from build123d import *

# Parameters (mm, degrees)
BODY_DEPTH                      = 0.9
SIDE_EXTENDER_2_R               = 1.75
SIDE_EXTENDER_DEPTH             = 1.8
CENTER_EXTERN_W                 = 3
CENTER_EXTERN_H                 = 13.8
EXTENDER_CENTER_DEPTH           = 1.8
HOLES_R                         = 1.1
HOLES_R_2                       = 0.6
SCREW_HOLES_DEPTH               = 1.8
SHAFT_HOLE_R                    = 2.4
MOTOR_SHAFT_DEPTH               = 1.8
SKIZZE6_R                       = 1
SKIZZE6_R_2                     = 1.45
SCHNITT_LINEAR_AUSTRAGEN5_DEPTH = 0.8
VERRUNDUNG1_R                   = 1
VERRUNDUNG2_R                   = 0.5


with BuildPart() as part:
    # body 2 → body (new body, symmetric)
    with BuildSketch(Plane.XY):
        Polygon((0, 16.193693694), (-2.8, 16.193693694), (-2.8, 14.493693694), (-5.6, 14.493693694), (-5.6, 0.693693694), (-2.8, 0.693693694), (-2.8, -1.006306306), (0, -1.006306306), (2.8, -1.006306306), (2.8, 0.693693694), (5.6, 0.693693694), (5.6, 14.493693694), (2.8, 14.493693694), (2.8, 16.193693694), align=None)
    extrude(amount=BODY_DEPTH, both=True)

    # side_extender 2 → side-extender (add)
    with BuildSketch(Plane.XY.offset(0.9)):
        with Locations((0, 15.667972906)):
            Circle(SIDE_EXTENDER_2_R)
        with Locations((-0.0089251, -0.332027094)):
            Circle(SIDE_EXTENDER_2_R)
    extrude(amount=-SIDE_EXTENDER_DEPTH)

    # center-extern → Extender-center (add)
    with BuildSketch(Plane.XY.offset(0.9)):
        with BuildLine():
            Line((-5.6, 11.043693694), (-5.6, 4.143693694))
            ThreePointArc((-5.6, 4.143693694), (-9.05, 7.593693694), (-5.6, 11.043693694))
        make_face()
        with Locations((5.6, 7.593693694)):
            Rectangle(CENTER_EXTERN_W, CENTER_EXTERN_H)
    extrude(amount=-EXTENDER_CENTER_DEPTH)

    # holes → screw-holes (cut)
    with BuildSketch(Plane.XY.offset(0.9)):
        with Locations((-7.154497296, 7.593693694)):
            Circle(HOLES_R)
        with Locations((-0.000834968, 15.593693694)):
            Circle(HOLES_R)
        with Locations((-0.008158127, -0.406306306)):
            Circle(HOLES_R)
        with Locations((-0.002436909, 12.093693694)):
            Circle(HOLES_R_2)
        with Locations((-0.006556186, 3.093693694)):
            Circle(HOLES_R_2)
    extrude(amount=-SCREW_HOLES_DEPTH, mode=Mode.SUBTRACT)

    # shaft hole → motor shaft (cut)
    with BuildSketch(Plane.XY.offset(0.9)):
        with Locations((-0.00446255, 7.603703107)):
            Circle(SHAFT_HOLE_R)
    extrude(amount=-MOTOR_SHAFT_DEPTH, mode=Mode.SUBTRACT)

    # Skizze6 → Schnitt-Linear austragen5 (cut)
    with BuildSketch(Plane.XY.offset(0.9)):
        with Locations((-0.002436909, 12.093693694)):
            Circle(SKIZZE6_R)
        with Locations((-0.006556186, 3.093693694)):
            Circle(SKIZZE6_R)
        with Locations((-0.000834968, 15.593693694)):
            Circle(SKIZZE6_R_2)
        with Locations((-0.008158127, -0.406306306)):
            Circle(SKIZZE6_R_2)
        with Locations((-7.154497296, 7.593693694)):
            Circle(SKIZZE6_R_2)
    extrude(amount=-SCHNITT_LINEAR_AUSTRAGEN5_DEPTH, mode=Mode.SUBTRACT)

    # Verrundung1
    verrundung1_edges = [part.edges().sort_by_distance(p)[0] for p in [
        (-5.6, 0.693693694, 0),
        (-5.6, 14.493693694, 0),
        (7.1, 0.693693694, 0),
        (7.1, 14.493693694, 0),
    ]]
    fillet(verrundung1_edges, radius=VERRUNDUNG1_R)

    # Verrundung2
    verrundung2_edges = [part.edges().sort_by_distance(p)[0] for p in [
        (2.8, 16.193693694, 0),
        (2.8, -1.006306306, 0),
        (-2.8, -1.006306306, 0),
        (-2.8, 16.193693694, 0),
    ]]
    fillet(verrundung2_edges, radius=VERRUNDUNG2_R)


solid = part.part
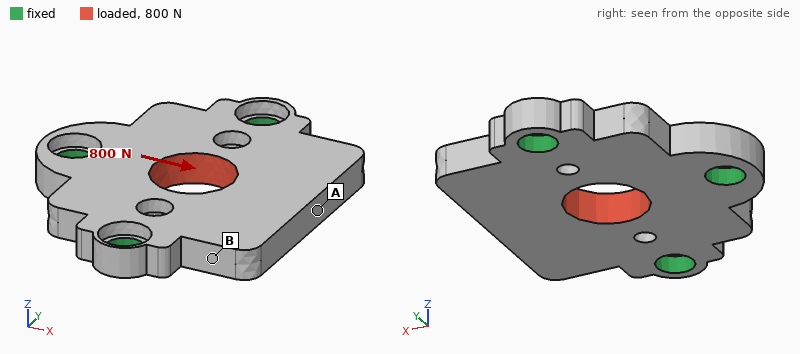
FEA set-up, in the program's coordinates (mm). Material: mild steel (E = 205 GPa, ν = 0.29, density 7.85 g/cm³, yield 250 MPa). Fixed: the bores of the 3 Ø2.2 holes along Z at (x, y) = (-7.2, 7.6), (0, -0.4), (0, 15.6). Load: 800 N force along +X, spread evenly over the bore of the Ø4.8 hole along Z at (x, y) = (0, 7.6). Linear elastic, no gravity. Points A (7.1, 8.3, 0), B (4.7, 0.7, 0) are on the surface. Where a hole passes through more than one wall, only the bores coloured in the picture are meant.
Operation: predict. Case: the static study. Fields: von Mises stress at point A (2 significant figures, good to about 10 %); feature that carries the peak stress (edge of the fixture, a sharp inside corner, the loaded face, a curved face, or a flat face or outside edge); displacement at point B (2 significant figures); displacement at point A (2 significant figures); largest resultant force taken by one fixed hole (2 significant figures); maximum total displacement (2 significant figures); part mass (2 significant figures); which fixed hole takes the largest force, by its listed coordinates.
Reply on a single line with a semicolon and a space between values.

42 MPa; edge of the fixture; 1.6 µm; 3.3 µm; 400 N; 3.5 µm; 2.5 g; (-7.2, 7.6)
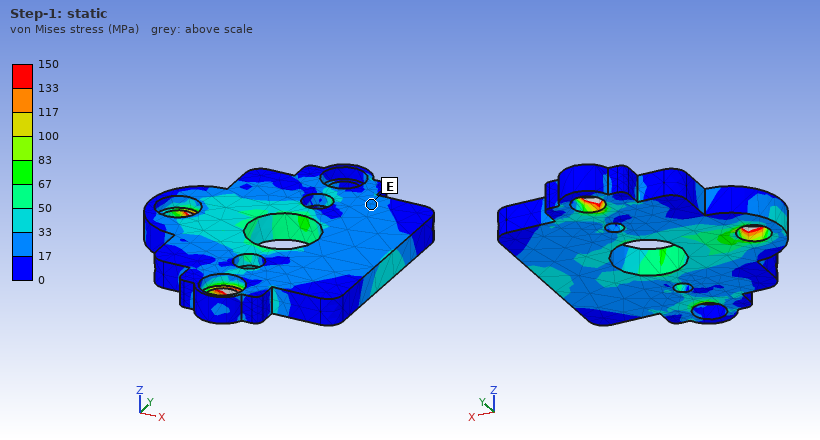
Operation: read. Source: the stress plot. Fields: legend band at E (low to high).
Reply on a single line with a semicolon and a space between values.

17 to 33 MPa
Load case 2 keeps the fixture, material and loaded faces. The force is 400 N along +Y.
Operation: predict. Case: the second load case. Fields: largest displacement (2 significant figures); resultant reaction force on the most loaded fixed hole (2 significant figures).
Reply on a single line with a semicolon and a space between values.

0.88 µm; 170 N
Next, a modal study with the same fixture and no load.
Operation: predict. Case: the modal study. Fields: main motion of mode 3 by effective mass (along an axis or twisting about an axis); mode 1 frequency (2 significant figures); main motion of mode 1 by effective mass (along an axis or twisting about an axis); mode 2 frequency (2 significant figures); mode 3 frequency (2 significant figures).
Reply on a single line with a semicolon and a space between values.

along Z; 17 kHz; along Z; 39 kHz; 53 kHz
